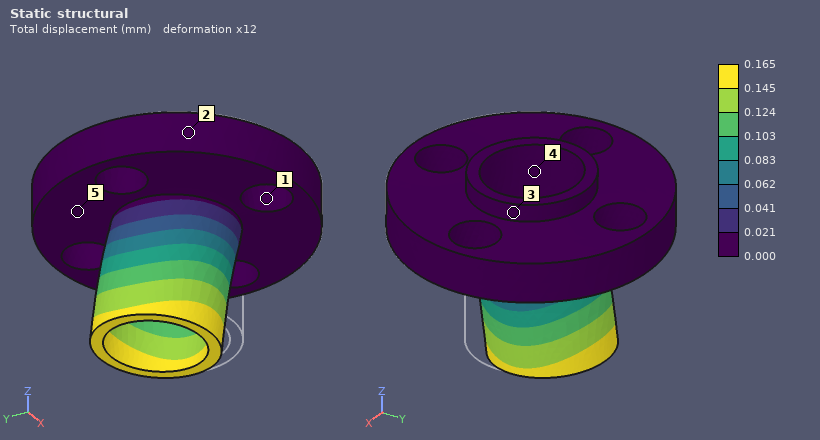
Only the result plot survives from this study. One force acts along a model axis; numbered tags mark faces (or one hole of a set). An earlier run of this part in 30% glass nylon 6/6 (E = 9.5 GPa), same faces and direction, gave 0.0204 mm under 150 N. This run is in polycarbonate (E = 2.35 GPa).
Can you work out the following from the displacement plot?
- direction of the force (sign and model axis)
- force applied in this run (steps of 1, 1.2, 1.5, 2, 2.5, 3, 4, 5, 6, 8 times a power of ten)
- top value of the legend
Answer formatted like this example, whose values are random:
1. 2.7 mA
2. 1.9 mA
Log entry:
1. +Y
2. 300 N
3. 0.165 mm
